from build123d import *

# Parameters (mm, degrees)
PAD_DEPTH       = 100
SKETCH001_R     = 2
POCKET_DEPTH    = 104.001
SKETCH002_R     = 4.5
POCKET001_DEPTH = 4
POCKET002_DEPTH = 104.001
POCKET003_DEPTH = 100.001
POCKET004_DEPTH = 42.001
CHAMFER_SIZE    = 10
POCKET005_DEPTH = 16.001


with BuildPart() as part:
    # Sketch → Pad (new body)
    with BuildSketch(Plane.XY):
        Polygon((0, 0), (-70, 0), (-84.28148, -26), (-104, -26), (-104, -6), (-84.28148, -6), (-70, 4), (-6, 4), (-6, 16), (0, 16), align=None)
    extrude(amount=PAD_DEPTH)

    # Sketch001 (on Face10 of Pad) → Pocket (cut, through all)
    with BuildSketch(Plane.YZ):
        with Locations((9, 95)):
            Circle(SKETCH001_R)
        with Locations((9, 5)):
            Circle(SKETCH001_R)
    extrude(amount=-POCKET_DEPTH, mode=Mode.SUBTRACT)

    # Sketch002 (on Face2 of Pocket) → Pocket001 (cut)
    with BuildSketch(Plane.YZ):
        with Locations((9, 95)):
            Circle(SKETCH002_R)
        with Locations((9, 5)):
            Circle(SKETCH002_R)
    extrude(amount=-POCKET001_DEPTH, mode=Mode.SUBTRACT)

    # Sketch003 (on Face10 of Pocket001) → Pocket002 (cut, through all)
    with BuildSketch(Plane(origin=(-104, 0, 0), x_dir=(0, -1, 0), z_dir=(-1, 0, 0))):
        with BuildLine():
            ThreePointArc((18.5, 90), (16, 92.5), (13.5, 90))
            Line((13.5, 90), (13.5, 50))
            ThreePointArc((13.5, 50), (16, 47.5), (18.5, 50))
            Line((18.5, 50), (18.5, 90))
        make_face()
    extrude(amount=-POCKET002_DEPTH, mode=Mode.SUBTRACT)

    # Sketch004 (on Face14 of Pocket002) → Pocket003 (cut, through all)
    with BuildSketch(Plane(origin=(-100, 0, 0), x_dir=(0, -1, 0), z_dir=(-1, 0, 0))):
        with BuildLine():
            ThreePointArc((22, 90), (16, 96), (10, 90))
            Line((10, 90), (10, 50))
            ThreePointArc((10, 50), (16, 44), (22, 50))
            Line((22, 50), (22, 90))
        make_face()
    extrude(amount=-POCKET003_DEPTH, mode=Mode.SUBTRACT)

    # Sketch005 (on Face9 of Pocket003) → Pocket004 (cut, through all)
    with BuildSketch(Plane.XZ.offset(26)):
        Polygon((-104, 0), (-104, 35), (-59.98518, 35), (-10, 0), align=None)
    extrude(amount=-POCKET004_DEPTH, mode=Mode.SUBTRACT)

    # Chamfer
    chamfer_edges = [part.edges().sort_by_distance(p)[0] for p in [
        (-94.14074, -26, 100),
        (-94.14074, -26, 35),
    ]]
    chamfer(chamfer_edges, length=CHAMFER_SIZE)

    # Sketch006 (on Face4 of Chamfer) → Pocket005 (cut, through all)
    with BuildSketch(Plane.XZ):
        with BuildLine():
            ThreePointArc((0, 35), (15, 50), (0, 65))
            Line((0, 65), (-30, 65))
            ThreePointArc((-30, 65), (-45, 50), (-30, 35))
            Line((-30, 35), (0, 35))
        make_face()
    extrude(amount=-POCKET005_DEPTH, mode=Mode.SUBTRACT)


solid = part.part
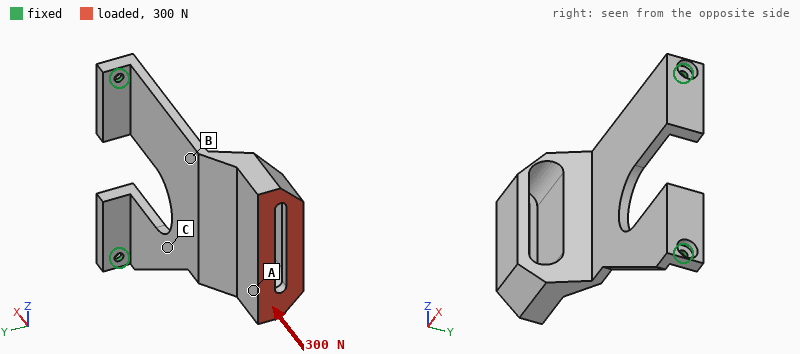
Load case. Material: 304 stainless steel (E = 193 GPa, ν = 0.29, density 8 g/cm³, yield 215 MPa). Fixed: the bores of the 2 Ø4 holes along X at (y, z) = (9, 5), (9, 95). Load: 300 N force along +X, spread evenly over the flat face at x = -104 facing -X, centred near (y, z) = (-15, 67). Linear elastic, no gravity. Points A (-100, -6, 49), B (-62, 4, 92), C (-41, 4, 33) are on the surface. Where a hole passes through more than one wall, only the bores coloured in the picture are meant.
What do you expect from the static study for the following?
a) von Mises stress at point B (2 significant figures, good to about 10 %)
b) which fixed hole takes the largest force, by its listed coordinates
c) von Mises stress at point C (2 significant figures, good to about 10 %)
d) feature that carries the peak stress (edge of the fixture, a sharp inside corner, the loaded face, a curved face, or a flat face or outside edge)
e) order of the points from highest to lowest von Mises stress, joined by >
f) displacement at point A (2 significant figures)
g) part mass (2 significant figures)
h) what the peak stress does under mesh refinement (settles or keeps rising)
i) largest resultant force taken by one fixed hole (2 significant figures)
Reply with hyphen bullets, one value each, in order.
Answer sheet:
- 28 MPa
- (9, 95)
- 44 MPa
- edge of the fixture
- C > B > A
- 0.54 mm
- 350 g
- keeps rising
- 220 N
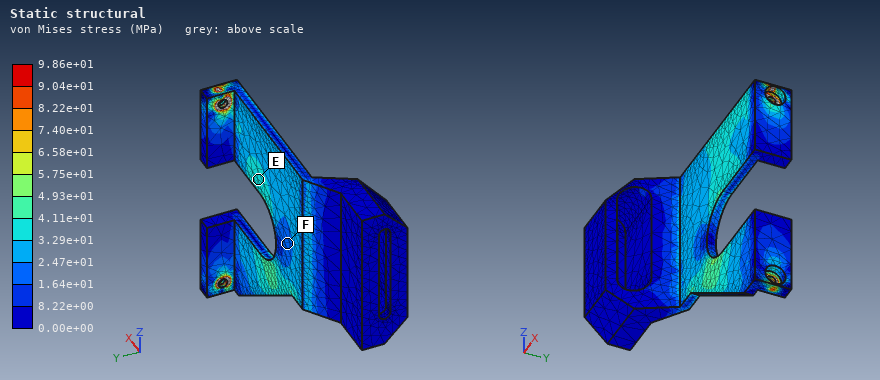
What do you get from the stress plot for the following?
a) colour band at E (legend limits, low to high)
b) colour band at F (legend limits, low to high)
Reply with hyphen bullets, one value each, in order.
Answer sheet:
- 3.29e+01 to 4.11e+01 MPa
- 1.64e+01 to 2.47e+01 MPa
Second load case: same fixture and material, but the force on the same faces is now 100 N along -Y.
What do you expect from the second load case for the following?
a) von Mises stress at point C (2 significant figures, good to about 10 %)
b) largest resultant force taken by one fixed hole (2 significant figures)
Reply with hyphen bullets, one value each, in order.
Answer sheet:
- 59 MPa
- 56 N
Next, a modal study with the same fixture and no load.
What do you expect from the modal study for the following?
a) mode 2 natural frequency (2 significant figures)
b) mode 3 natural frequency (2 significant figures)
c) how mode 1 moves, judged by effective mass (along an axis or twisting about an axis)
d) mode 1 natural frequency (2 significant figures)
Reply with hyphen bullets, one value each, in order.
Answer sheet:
- 650 Hz
- 1100 Hz
- along Y
- 150 Hz
